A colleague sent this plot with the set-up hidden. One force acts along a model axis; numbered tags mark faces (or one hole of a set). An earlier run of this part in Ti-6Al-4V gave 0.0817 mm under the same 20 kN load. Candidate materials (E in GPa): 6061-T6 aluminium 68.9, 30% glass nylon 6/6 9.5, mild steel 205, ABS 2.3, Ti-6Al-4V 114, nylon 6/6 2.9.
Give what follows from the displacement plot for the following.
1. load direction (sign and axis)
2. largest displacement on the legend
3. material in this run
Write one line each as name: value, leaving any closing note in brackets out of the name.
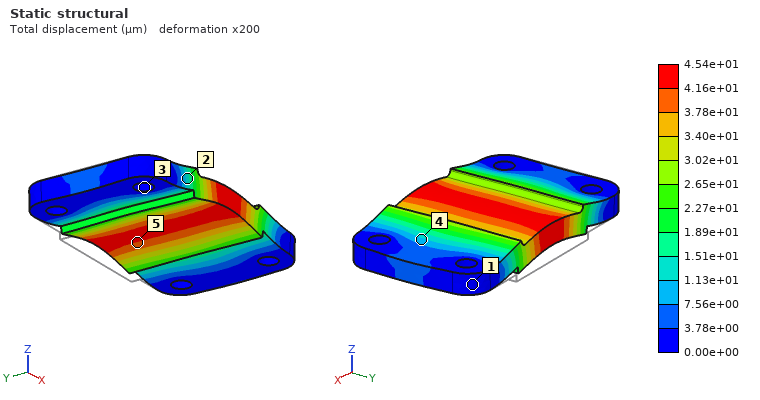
load direction: +Z
largest displacement on the legend: 4.54e+01 µm
material in this run: mild steel
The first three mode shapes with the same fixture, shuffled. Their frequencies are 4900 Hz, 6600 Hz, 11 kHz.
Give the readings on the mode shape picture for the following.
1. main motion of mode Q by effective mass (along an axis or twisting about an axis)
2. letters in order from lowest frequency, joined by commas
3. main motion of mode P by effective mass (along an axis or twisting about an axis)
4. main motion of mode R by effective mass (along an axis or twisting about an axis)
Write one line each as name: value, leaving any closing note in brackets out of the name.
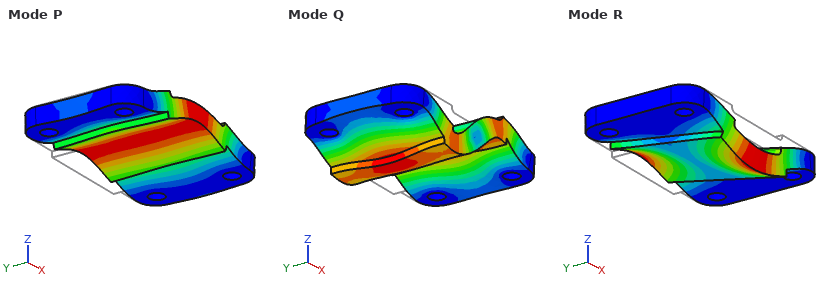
main motion of mode Q by effective mass: twisting about Y
letters in order from lowest frequency, joined by commas: P, R, Q
main motion of mode P by effective mass: along Z
main motion of mode R by effective mass: twisting about X
